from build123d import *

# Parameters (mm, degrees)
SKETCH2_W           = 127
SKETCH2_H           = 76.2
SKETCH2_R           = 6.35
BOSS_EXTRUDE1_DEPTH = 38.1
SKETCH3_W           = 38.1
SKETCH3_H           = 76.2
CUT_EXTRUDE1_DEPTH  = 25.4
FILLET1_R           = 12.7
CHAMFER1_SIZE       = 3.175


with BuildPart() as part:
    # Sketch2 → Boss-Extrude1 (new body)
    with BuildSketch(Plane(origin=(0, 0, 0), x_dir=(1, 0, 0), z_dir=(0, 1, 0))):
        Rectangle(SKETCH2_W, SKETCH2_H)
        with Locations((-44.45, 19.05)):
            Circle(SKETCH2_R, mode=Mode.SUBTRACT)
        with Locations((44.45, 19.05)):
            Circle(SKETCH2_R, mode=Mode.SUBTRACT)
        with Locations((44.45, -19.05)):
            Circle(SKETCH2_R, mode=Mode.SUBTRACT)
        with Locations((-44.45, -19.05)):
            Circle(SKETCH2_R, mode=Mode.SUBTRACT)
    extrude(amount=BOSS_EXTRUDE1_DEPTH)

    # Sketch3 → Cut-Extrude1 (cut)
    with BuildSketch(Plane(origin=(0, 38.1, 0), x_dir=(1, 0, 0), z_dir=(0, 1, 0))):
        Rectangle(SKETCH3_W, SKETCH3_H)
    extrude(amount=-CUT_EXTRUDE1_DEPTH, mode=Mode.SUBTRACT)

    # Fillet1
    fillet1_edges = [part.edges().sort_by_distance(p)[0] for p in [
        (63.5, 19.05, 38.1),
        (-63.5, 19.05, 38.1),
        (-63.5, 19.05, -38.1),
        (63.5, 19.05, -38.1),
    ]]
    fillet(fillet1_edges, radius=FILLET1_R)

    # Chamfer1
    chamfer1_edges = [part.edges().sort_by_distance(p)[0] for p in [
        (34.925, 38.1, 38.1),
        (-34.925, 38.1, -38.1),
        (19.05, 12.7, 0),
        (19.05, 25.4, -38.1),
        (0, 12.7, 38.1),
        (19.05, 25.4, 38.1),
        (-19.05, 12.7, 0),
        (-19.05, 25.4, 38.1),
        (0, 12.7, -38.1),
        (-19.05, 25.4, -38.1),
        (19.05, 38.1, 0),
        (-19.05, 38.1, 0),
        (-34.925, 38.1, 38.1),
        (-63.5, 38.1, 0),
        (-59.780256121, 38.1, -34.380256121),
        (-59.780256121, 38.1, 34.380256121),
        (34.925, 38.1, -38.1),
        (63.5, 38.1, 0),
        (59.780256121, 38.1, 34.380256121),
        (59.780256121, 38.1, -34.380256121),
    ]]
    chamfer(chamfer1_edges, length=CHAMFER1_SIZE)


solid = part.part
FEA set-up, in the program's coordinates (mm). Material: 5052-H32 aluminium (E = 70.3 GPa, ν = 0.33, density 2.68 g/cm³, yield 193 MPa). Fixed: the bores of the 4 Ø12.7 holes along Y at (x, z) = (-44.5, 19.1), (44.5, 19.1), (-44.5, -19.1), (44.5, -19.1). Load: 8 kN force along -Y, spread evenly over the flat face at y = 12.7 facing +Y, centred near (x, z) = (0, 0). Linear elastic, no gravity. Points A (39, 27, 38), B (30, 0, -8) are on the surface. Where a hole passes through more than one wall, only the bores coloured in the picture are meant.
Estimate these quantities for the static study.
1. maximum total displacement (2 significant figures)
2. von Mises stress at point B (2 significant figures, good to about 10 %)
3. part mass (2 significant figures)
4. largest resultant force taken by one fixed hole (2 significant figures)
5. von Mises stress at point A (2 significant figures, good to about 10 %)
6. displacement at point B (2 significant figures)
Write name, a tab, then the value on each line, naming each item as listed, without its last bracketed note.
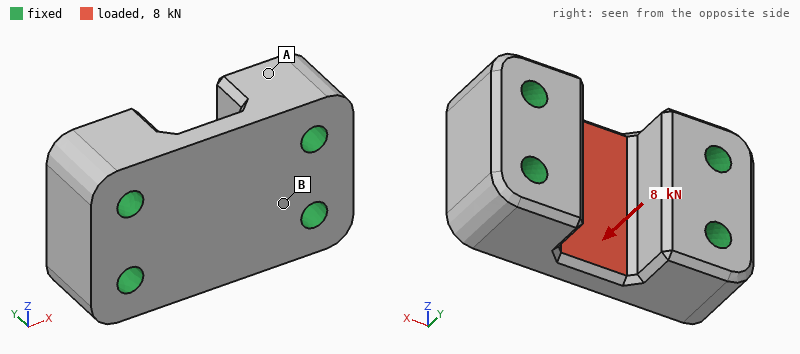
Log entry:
maximum total displacement	8.0 µm
von Mises stress at point B	4.6 MPa
part mass	720 g
largest resultant force taken by one fixed hole	2.2 kN
von Mises stress at point A	1.9 MPa
displacement at point B	1.7 µm
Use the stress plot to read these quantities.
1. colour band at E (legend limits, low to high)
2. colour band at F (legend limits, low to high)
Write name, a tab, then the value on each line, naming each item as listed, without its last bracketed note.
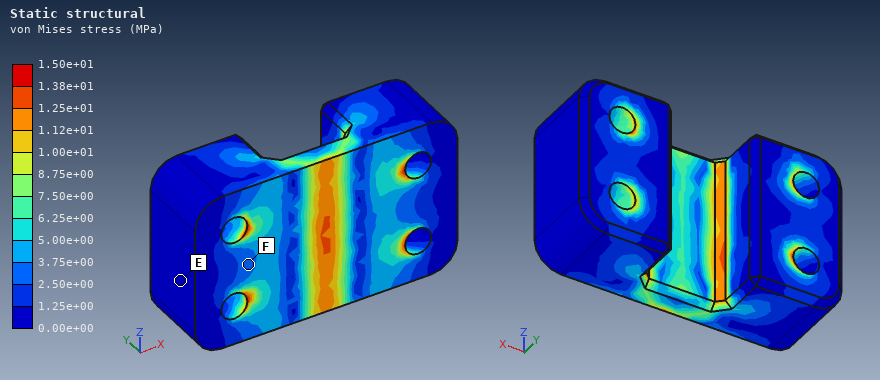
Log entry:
colour band at E	0.00e+00 to 1.25e+00 MPa
colour band at F	2.50e+00 to 3.75e+00 MPa
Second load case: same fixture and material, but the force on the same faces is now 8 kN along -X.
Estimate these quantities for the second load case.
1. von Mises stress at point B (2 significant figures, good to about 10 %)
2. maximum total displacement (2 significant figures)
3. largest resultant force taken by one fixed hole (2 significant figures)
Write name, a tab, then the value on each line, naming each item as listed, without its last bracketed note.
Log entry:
von Mises stress at point B	3.3 MPa
maximum total displacement	3.0 µm
largest resultant force taken by one fixed hole	2.1 kN
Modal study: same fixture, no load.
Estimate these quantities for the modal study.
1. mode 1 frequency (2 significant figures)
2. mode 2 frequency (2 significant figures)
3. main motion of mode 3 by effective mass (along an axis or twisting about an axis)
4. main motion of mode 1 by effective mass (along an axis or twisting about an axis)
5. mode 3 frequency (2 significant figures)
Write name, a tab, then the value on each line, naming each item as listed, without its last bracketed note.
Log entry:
mode 1 frequency	17 kHz
mode 2 frequency	18 kHz
main motion of mode 3 by effective mass	along Z
main motion of mode 1 by effective mass	along Y
mode 3 frequency	20 kHz
